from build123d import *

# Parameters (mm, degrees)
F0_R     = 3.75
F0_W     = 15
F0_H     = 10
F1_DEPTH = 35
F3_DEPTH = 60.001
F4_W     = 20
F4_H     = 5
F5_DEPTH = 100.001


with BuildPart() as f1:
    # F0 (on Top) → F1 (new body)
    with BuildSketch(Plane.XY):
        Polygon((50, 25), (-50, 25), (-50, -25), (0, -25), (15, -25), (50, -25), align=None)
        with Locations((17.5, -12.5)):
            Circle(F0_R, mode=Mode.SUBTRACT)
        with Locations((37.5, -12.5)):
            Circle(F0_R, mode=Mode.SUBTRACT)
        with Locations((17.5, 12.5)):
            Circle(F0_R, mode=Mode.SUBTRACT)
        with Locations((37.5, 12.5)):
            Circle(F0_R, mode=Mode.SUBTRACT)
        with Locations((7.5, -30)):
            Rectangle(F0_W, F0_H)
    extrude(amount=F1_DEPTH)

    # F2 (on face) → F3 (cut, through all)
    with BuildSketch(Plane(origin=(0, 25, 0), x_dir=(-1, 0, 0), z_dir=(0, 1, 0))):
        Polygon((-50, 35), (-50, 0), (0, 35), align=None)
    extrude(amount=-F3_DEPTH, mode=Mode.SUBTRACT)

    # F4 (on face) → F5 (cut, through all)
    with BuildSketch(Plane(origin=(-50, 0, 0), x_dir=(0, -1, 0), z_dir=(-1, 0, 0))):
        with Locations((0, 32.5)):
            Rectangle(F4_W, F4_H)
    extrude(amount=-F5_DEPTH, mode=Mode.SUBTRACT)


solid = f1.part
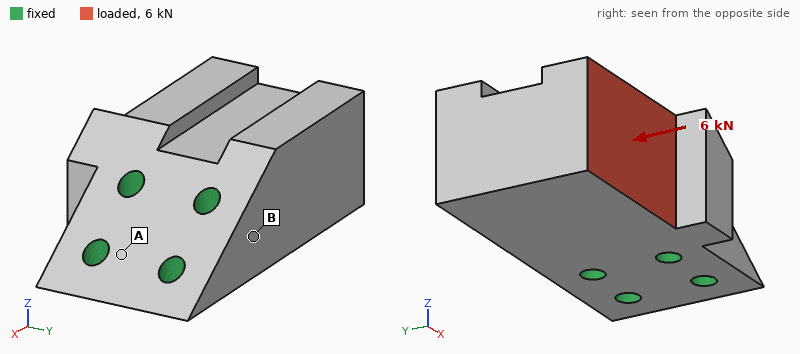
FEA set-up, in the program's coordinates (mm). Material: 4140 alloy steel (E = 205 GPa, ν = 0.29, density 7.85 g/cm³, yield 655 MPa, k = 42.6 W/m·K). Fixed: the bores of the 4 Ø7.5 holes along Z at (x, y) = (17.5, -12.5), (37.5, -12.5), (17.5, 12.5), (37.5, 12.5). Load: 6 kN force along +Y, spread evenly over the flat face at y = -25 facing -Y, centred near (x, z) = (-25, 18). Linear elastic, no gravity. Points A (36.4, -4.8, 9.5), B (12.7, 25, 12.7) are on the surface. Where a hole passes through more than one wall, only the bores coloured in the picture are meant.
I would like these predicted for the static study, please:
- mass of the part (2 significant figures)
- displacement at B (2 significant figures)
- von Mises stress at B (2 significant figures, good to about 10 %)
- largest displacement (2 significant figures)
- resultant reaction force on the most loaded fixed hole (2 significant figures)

1.0 kg
1.6 µm
14 MPa
10 µm
7.9 kN
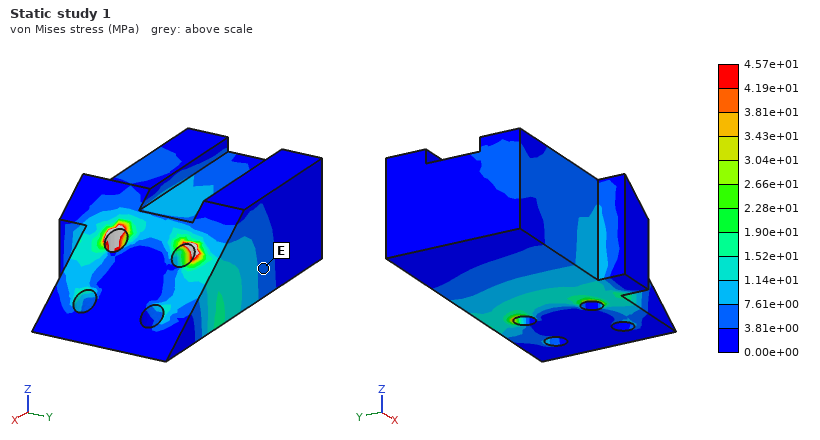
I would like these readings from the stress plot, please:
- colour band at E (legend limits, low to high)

3.81e+00 to 7.61e+00 MPa
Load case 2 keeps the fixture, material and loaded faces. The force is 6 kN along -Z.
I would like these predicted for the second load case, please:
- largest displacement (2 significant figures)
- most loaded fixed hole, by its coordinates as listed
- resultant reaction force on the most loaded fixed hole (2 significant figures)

29 µm
(17.5, -12.5)
6.5 kN
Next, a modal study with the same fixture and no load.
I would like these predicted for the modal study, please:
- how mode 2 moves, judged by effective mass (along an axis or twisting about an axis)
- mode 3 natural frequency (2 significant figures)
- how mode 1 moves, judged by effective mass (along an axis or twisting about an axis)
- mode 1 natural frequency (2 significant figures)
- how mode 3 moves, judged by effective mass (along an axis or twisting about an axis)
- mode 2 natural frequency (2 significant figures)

along Y
9000 Hz
along Z
3900 Hz
twisting about X
5800 Hz
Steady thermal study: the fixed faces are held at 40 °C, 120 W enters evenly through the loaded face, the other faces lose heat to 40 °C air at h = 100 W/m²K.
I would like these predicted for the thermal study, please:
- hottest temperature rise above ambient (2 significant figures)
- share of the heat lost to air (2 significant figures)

77 K
35 %
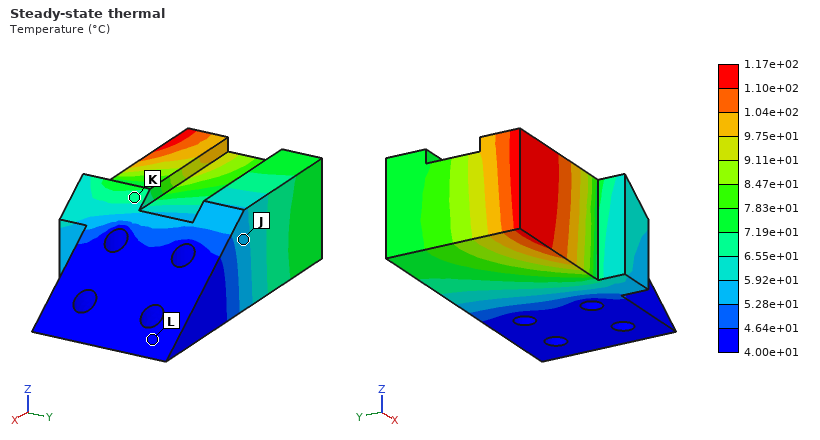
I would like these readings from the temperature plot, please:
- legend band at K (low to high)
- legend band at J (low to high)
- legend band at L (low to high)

6.55e+01 to 7.19e+01 °C
5.28e+01 to 5.92e+01 °C
4.00e+01 to 4.64e+01 °C
